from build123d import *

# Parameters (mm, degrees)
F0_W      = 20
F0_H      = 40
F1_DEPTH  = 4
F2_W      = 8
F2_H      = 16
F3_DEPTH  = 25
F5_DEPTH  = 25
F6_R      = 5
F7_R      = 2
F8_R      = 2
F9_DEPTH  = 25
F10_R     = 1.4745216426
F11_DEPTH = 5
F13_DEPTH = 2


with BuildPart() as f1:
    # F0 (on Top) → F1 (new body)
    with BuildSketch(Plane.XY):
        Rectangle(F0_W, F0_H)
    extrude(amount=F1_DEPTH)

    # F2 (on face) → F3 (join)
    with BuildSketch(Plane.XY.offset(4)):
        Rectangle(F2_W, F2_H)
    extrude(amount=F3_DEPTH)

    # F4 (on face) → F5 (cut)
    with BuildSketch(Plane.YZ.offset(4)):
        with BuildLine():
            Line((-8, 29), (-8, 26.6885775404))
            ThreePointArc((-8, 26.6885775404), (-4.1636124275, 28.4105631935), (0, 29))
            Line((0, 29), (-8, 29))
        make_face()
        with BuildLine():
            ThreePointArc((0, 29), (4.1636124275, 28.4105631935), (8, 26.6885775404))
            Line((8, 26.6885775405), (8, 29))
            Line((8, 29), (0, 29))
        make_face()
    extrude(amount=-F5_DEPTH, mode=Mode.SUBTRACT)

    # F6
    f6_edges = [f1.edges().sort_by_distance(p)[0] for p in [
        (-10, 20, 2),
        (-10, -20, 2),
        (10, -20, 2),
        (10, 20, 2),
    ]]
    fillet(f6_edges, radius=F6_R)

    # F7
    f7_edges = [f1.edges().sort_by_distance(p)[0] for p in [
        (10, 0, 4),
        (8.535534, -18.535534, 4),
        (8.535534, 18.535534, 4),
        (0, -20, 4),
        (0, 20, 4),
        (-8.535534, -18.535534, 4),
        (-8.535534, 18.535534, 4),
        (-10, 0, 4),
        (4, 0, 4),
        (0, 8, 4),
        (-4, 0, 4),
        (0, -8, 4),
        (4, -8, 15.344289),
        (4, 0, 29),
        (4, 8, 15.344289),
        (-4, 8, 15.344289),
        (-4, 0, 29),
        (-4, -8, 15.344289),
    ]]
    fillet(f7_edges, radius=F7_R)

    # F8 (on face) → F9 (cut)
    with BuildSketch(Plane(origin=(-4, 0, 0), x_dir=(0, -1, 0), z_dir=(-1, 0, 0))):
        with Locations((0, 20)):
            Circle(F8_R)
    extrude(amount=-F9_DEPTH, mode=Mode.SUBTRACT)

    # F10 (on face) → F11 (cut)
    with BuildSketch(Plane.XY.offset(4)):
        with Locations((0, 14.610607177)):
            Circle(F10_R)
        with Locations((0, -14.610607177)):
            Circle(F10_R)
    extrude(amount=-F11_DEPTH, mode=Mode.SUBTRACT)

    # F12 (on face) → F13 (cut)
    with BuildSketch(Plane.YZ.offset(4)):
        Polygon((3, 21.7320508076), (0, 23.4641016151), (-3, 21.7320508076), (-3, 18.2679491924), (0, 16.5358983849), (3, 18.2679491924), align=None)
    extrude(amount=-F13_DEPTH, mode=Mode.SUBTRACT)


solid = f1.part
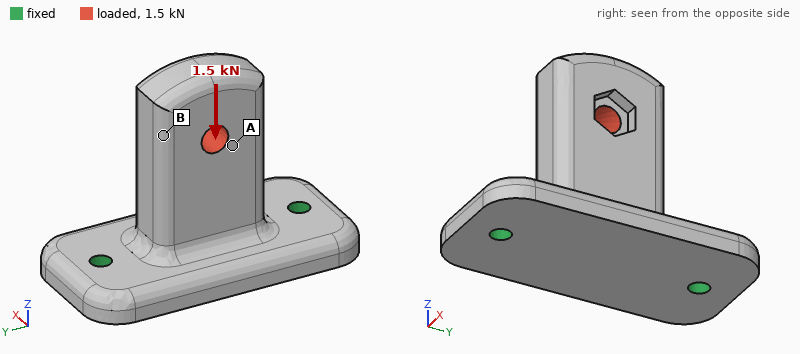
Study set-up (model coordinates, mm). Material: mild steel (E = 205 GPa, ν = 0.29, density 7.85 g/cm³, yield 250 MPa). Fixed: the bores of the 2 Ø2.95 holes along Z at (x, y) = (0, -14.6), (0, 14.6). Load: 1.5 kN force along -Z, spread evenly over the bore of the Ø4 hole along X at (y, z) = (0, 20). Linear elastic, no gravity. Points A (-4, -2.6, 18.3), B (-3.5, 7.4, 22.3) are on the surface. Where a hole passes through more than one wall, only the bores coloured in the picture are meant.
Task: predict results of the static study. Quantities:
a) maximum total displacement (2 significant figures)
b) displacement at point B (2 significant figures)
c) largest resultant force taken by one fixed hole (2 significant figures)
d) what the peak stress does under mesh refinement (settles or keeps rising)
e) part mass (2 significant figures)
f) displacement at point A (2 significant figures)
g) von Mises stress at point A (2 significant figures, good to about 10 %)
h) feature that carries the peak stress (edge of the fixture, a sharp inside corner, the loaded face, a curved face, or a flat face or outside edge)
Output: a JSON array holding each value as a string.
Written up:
["11 µm", "9.2 µm", "800 N", "keeps rising", "46 g", "8.5 µm", "27 MPa", "edge of the fixture"]
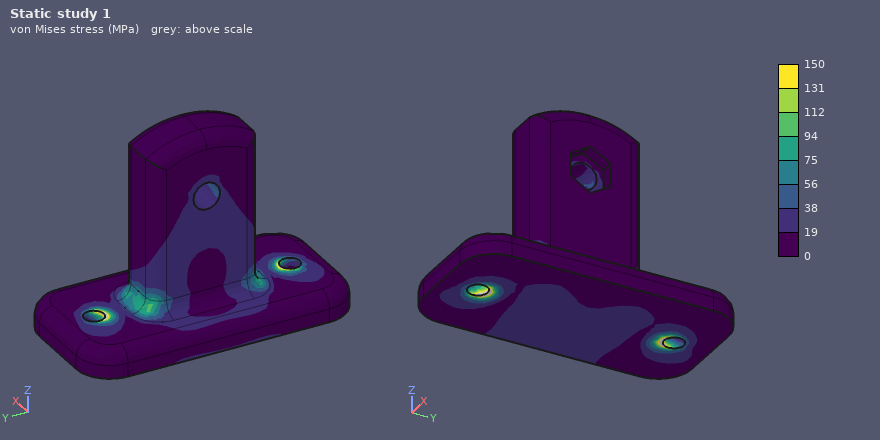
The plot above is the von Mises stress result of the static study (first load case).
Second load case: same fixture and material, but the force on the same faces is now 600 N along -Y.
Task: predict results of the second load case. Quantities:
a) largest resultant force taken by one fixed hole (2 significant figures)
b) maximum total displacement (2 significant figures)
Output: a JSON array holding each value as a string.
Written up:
["550 N", "9.8 µm"]
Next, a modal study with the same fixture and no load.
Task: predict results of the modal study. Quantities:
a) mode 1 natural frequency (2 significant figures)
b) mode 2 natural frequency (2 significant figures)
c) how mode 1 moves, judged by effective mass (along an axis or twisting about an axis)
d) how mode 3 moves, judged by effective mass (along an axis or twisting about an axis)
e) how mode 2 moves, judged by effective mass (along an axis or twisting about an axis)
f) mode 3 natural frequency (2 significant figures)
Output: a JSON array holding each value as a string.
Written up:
["4800 Hz", "11 kHz", "along X", "along Z", "along Y", "15 kHz"]
